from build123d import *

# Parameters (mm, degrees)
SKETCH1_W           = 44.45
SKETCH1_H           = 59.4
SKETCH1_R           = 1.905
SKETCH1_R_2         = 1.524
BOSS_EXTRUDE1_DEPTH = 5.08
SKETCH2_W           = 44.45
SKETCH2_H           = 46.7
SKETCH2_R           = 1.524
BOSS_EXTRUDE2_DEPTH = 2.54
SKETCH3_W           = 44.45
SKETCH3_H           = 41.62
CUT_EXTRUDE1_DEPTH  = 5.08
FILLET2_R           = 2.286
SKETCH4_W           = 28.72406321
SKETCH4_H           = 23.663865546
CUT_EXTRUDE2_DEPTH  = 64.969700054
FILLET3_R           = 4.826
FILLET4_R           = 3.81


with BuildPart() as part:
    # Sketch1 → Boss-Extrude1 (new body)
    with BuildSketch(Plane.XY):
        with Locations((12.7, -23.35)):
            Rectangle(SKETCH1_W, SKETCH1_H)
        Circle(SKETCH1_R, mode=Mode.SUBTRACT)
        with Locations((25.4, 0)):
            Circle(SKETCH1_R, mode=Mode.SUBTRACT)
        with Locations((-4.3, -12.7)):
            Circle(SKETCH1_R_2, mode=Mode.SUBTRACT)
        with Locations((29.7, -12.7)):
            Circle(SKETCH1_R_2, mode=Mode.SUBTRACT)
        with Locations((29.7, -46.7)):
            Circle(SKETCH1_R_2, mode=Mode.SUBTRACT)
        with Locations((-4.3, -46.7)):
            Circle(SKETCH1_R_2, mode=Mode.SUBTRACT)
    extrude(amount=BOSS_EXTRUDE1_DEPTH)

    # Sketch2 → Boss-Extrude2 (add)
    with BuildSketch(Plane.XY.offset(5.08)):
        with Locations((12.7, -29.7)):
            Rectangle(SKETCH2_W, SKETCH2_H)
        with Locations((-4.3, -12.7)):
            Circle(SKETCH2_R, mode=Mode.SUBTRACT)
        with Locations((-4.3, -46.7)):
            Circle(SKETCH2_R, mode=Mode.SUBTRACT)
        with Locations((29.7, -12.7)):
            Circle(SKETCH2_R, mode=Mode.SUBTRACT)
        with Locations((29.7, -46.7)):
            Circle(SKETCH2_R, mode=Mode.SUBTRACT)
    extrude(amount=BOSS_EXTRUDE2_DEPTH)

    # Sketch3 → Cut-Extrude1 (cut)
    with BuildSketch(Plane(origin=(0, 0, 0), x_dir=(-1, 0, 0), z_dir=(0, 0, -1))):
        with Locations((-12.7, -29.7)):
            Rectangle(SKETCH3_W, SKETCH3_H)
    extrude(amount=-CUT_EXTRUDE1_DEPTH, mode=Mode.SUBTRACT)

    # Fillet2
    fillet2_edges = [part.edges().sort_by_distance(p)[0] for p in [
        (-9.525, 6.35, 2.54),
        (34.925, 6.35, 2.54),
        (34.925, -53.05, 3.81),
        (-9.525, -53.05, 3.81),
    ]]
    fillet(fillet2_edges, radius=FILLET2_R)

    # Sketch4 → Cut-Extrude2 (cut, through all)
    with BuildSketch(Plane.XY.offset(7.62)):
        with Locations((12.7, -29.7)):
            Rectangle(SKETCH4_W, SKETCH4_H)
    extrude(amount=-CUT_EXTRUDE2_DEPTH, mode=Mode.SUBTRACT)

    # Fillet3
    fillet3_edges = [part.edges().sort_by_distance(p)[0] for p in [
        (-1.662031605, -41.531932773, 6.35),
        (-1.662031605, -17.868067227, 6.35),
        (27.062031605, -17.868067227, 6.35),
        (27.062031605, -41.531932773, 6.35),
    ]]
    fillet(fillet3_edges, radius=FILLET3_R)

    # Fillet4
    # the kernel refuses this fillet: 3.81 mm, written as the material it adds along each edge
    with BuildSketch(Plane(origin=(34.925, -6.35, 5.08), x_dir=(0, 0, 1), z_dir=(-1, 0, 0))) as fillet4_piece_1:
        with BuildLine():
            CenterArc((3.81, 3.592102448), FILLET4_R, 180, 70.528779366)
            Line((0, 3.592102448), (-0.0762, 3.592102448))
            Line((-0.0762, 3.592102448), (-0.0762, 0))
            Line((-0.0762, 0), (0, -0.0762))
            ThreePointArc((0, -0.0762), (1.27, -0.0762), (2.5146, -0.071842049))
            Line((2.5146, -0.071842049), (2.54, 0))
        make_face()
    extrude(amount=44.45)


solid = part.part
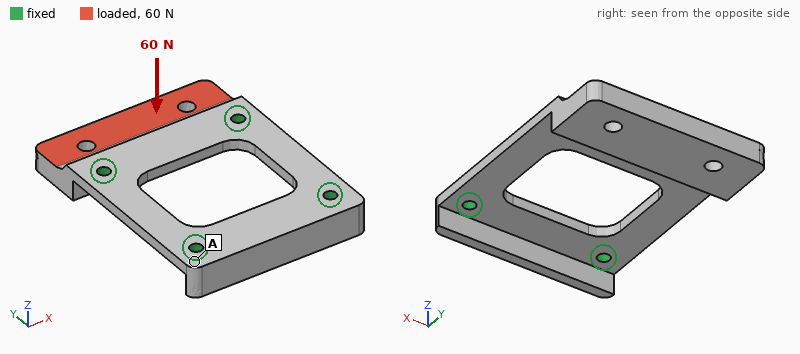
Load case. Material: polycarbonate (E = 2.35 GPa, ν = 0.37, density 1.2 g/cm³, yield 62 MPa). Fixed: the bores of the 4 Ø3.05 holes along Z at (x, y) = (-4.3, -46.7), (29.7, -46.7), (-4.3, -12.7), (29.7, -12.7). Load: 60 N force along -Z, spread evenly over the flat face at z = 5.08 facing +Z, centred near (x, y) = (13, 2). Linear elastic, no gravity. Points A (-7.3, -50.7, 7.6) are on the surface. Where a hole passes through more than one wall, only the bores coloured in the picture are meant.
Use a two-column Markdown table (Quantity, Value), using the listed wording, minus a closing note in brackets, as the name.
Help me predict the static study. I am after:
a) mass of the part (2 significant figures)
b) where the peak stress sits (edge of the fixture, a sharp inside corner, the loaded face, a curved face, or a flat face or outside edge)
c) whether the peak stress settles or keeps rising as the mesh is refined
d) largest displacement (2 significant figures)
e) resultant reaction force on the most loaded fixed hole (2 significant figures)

| Quantity | Value |
|---|---|
| mass of the part | 9.0 g |
| where the peak stress sits | edge of the fixture |
| whether the peak stress settles or keeps rising as the mesh is refined | keeps rising |
| largest displacement | 0.68 mm |
| resultant reaction force on the most loaded fixed hole | 34 N |
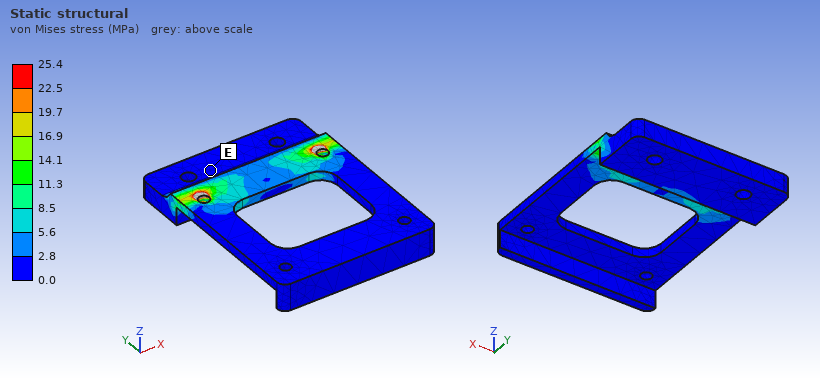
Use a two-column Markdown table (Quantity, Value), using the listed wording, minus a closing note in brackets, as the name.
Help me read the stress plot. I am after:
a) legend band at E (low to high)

| Quantity | Value |
|---|---|
| legend band at E | 0.0 to 2.8 MPa |
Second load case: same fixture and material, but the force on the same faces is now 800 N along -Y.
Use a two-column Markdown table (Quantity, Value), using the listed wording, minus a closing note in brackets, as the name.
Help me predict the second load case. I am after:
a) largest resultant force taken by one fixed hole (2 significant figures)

| Quantity | Value |
|---|---|
| largest resultant force taken by one fixed hole | 400 N |
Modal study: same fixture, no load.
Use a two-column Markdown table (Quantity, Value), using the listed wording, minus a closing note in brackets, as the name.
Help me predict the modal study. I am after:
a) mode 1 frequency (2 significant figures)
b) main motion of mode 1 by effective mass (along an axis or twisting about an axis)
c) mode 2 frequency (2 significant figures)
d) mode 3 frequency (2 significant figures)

| Quantity | Value |
|---|---|
| mode 1 frequency | 1000 Hz |
| main motion of mode 1 by effective mass | along Z |
| mode 2 frequency | 2700 Hz |
| mode 3 frequency | 3500 Hz |
